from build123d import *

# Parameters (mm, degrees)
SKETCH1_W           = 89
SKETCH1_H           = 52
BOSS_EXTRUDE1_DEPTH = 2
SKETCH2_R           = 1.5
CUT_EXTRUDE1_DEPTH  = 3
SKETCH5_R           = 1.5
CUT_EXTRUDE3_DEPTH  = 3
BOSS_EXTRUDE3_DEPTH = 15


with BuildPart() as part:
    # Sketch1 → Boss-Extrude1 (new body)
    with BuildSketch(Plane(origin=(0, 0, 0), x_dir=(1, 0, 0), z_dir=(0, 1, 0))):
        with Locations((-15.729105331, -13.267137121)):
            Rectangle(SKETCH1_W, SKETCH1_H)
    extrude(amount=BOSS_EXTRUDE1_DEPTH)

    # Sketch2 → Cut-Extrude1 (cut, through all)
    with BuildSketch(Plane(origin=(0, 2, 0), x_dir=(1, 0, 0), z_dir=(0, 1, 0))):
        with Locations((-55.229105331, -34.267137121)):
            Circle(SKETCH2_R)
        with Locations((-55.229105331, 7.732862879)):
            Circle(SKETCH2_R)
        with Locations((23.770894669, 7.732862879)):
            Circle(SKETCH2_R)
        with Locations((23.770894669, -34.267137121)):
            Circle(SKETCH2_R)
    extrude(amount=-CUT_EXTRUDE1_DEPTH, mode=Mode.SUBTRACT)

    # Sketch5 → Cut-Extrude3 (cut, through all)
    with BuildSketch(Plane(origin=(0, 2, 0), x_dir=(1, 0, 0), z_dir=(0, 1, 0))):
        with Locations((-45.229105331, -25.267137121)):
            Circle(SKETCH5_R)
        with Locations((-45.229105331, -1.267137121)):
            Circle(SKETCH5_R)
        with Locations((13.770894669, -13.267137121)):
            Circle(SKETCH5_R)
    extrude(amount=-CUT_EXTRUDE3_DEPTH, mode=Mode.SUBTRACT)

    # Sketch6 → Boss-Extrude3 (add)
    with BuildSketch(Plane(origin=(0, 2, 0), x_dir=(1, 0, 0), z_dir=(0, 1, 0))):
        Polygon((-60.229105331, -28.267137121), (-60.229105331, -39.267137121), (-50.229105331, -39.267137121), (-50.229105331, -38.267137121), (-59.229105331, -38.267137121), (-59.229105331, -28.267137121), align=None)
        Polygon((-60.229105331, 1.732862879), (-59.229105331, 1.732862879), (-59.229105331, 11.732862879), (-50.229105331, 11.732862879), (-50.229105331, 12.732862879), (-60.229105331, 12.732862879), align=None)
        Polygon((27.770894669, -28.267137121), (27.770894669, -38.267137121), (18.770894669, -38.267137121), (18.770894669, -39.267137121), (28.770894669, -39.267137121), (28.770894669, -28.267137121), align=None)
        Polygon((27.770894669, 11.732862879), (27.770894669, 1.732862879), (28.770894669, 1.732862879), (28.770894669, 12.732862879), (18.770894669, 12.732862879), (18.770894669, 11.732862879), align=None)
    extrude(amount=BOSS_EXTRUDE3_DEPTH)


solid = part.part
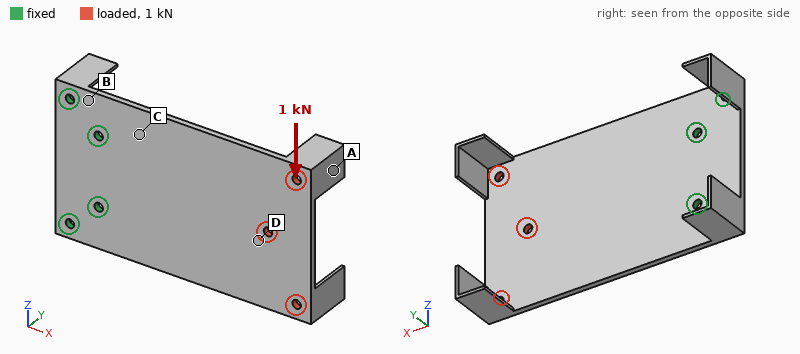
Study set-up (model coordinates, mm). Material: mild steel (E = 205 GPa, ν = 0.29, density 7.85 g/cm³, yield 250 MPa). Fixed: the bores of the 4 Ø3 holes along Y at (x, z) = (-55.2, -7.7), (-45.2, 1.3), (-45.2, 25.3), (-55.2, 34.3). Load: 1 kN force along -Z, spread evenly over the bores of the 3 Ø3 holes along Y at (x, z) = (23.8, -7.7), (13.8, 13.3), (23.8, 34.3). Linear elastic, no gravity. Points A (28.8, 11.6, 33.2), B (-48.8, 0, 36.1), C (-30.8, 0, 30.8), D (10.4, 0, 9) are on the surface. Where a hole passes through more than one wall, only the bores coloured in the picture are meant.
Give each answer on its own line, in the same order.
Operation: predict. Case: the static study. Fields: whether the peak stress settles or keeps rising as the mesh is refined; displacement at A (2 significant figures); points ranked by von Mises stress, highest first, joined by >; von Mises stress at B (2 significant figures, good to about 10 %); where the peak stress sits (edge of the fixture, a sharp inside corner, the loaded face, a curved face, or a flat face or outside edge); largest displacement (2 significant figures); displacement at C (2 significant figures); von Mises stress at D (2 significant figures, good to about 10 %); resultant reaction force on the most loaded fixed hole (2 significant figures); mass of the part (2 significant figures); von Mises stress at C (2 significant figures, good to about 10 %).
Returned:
keeps rising
42 µm
B > C > D > A
56 MPa
edge of the fixture
44 µm
7.1 µm
25 MPa
1.2 kN
81 g
40 MPa
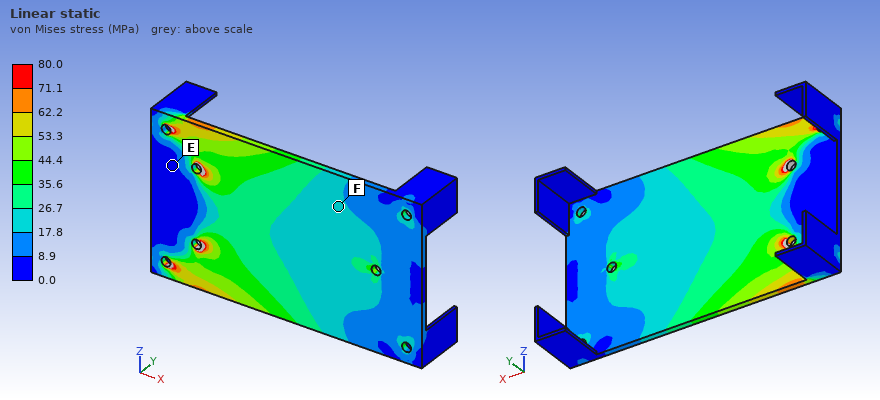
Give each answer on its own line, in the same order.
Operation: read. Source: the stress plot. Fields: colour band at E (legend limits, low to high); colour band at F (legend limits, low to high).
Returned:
0.0 to 8.9 MPa
17.8 to 26.7 MPa
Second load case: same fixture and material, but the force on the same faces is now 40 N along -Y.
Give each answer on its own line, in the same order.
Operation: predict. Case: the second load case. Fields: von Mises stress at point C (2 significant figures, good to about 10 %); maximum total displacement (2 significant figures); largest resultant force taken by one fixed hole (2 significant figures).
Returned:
56 MPa
0.65 mm
65 N
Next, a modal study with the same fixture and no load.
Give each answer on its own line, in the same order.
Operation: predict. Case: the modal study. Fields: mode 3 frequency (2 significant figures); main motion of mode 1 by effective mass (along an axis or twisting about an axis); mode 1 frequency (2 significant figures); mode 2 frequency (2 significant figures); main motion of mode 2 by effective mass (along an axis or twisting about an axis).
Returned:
1600 Hz
along Y
270 Hz
770 Hz
twisting about X
